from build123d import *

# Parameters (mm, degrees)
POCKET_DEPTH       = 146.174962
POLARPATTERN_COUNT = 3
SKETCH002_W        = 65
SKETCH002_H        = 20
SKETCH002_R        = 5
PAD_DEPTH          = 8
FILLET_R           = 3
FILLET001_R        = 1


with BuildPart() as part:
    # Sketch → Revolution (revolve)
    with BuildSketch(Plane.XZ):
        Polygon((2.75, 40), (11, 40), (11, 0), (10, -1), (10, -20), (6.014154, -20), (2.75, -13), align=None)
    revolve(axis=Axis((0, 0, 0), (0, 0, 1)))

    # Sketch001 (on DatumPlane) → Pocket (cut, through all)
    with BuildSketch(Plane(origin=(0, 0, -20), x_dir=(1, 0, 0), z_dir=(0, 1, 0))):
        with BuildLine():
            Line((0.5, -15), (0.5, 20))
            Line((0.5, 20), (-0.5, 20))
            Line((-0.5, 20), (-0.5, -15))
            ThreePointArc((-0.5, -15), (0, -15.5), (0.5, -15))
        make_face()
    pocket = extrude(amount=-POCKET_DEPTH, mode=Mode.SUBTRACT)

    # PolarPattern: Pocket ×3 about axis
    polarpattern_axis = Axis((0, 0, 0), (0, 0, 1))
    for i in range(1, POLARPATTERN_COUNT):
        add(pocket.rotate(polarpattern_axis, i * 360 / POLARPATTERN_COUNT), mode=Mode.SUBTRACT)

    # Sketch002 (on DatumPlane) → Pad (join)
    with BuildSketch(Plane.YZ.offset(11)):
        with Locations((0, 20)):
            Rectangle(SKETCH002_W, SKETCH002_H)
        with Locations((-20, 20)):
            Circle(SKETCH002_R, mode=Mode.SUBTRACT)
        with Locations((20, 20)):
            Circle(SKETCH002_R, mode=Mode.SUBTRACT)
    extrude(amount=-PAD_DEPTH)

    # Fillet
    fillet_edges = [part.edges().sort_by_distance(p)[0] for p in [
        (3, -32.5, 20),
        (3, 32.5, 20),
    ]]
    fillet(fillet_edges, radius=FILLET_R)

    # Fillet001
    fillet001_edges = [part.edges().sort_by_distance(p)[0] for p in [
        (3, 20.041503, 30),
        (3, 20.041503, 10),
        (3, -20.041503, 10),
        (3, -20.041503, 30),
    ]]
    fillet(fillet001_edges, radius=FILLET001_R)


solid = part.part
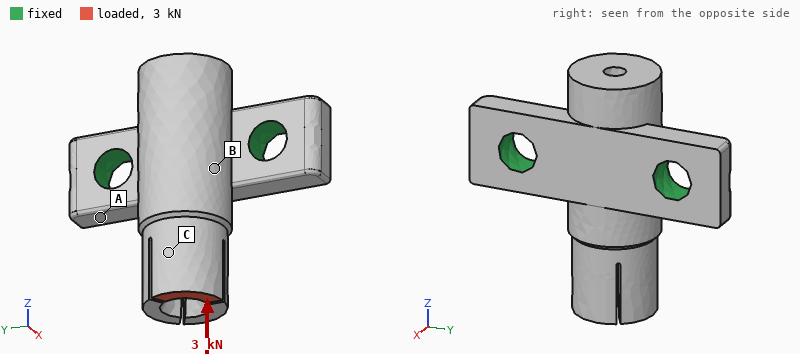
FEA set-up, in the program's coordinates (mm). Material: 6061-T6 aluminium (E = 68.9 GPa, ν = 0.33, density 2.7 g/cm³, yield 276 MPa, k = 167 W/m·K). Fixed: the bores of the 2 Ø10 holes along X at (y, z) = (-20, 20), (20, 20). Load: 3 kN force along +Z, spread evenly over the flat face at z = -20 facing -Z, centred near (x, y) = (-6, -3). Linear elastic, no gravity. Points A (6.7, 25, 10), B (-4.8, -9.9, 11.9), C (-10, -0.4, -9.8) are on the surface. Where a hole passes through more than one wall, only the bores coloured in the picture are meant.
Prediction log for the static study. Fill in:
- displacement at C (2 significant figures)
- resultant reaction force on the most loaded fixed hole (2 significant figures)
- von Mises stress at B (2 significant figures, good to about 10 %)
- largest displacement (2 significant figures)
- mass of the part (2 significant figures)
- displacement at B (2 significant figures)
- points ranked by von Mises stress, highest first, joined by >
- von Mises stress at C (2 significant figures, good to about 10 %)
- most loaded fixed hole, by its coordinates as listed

0.090 mm
1.8 kN
26 MPa
0.13 mm
70 g
0.034 mm
C > B > A
57 MPa
(-20, 20)
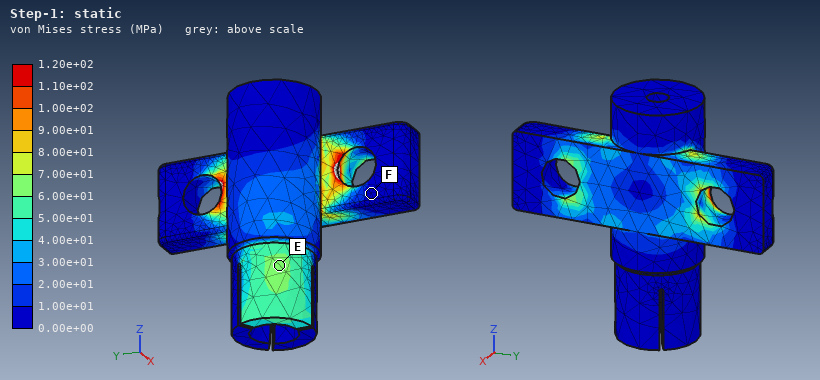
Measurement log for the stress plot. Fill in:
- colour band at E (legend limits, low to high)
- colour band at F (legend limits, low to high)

6.00e+01 to 7.00e+01 MPa
0.00e+00 to 1.00e+01 MPa
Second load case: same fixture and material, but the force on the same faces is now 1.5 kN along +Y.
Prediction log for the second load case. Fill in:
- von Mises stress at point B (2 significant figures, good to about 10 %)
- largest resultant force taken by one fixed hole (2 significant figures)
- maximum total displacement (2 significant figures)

32 MPa
2.0 kN
0.14 mm
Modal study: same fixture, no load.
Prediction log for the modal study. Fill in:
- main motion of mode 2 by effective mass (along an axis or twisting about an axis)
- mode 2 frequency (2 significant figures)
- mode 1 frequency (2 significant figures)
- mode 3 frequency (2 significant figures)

along Y
9200 Hz
4500 Hz
14 kHz
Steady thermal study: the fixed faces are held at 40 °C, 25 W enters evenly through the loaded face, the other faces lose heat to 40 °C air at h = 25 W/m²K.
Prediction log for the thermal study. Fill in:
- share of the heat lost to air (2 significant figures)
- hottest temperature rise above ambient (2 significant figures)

6.1 %
46 K
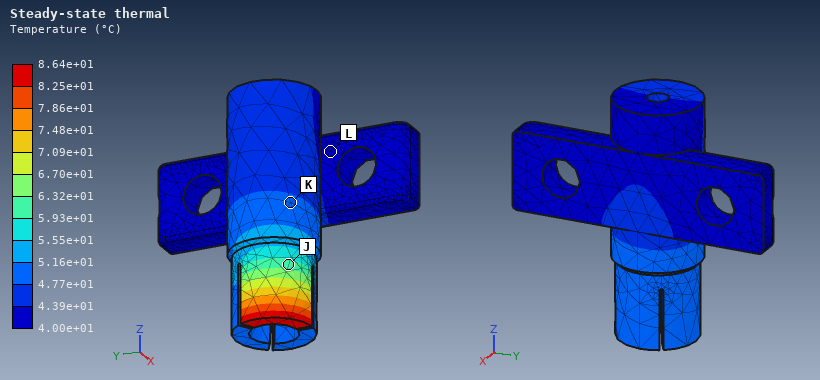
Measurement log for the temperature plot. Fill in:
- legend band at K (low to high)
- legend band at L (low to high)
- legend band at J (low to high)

4.77e+01 to 5.16e+01 °C
4.00e+01 to 4.39e+01 °C
5.93e+01 to 6.32e+01 °C
